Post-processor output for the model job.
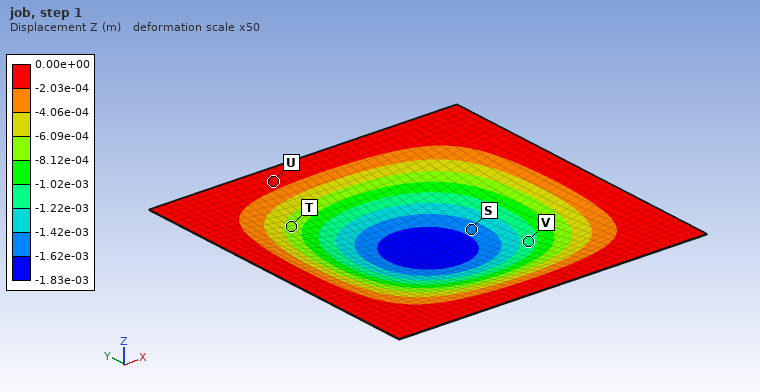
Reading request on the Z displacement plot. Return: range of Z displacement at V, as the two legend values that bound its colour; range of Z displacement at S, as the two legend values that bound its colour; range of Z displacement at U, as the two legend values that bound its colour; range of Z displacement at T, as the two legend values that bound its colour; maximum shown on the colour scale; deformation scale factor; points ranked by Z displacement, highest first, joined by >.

-1.22e-03 to -1.02e-03 m
-1.62e-03 to -1.42e-03 m
-2.03e-04 to 0.00e+00 m
-8.12e-04 to -6.09e-04 m
0.00e+00 m
50
U > T > V > S
